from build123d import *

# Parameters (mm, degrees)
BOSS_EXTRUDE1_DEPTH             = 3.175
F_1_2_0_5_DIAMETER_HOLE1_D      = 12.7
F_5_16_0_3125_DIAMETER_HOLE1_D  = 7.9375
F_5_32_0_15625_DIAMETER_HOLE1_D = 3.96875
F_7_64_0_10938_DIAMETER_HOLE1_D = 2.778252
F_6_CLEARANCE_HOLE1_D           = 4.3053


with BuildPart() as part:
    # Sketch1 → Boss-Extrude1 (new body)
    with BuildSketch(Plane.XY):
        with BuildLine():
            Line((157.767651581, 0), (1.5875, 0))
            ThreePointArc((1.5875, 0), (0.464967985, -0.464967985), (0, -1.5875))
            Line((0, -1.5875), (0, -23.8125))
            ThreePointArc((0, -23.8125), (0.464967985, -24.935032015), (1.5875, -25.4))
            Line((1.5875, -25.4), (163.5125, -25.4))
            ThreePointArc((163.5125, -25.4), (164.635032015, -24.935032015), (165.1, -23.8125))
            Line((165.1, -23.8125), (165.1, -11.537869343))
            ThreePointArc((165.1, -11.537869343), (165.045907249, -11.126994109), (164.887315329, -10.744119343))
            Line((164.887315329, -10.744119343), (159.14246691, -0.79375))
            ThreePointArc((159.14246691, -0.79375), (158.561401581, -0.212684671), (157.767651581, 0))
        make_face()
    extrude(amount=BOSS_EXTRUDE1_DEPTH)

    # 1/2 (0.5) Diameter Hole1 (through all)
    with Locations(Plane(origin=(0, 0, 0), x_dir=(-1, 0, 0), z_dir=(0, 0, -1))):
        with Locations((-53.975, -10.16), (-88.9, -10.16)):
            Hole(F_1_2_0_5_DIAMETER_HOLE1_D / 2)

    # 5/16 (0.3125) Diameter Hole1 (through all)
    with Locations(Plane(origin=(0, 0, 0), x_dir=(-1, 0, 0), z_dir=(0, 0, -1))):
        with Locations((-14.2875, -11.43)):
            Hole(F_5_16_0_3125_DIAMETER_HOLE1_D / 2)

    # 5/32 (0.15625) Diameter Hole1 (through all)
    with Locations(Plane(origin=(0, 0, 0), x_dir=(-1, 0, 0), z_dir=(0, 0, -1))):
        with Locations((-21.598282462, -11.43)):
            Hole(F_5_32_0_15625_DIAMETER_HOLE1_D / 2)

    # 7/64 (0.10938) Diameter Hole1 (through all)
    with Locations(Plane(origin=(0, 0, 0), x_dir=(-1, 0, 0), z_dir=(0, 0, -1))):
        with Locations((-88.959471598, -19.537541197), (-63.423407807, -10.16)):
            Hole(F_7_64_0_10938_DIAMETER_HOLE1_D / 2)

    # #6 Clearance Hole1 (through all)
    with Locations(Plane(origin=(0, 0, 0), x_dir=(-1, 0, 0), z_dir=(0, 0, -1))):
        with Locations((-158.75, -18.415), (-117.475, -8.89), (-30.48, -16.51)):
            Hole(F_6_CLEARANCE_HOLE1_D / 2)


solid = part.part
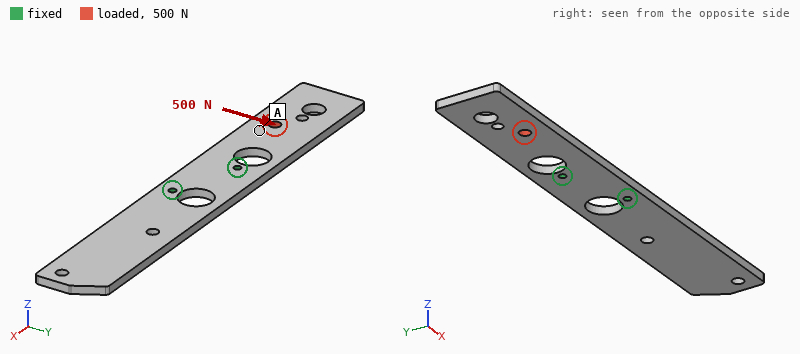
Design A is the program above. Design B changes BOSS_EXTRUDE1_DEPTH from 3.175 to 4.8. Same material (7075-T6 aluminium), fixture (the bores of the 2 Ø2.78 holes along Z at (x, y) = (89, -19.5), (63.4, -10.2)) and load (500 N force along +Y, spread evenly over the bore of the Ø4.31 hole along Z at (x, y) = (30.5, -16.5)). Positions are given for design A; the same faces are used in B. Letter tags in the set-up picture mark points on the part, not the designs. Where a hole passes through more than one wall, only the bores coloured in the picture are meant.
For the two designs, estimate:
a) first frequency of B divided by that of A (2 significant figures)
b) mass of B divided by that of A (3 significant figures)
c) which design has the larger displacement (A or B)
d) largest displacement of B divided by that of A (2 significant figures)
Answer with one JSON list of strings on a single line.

["1.5", "1.51", "A", "0.66"]
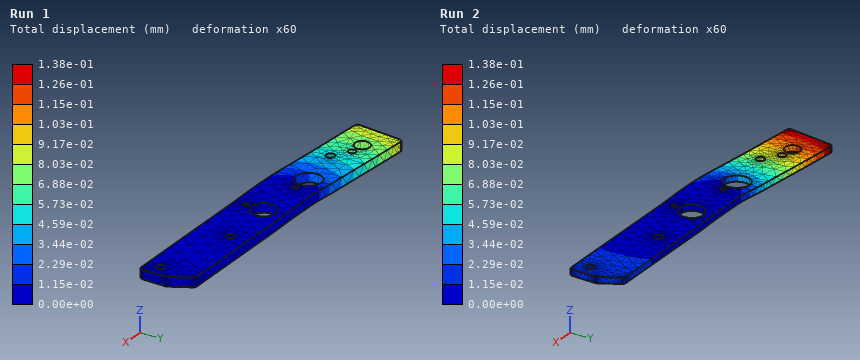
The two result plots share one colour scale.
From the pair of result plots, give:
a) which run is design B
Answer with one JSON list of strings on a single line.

["Run 1"]
